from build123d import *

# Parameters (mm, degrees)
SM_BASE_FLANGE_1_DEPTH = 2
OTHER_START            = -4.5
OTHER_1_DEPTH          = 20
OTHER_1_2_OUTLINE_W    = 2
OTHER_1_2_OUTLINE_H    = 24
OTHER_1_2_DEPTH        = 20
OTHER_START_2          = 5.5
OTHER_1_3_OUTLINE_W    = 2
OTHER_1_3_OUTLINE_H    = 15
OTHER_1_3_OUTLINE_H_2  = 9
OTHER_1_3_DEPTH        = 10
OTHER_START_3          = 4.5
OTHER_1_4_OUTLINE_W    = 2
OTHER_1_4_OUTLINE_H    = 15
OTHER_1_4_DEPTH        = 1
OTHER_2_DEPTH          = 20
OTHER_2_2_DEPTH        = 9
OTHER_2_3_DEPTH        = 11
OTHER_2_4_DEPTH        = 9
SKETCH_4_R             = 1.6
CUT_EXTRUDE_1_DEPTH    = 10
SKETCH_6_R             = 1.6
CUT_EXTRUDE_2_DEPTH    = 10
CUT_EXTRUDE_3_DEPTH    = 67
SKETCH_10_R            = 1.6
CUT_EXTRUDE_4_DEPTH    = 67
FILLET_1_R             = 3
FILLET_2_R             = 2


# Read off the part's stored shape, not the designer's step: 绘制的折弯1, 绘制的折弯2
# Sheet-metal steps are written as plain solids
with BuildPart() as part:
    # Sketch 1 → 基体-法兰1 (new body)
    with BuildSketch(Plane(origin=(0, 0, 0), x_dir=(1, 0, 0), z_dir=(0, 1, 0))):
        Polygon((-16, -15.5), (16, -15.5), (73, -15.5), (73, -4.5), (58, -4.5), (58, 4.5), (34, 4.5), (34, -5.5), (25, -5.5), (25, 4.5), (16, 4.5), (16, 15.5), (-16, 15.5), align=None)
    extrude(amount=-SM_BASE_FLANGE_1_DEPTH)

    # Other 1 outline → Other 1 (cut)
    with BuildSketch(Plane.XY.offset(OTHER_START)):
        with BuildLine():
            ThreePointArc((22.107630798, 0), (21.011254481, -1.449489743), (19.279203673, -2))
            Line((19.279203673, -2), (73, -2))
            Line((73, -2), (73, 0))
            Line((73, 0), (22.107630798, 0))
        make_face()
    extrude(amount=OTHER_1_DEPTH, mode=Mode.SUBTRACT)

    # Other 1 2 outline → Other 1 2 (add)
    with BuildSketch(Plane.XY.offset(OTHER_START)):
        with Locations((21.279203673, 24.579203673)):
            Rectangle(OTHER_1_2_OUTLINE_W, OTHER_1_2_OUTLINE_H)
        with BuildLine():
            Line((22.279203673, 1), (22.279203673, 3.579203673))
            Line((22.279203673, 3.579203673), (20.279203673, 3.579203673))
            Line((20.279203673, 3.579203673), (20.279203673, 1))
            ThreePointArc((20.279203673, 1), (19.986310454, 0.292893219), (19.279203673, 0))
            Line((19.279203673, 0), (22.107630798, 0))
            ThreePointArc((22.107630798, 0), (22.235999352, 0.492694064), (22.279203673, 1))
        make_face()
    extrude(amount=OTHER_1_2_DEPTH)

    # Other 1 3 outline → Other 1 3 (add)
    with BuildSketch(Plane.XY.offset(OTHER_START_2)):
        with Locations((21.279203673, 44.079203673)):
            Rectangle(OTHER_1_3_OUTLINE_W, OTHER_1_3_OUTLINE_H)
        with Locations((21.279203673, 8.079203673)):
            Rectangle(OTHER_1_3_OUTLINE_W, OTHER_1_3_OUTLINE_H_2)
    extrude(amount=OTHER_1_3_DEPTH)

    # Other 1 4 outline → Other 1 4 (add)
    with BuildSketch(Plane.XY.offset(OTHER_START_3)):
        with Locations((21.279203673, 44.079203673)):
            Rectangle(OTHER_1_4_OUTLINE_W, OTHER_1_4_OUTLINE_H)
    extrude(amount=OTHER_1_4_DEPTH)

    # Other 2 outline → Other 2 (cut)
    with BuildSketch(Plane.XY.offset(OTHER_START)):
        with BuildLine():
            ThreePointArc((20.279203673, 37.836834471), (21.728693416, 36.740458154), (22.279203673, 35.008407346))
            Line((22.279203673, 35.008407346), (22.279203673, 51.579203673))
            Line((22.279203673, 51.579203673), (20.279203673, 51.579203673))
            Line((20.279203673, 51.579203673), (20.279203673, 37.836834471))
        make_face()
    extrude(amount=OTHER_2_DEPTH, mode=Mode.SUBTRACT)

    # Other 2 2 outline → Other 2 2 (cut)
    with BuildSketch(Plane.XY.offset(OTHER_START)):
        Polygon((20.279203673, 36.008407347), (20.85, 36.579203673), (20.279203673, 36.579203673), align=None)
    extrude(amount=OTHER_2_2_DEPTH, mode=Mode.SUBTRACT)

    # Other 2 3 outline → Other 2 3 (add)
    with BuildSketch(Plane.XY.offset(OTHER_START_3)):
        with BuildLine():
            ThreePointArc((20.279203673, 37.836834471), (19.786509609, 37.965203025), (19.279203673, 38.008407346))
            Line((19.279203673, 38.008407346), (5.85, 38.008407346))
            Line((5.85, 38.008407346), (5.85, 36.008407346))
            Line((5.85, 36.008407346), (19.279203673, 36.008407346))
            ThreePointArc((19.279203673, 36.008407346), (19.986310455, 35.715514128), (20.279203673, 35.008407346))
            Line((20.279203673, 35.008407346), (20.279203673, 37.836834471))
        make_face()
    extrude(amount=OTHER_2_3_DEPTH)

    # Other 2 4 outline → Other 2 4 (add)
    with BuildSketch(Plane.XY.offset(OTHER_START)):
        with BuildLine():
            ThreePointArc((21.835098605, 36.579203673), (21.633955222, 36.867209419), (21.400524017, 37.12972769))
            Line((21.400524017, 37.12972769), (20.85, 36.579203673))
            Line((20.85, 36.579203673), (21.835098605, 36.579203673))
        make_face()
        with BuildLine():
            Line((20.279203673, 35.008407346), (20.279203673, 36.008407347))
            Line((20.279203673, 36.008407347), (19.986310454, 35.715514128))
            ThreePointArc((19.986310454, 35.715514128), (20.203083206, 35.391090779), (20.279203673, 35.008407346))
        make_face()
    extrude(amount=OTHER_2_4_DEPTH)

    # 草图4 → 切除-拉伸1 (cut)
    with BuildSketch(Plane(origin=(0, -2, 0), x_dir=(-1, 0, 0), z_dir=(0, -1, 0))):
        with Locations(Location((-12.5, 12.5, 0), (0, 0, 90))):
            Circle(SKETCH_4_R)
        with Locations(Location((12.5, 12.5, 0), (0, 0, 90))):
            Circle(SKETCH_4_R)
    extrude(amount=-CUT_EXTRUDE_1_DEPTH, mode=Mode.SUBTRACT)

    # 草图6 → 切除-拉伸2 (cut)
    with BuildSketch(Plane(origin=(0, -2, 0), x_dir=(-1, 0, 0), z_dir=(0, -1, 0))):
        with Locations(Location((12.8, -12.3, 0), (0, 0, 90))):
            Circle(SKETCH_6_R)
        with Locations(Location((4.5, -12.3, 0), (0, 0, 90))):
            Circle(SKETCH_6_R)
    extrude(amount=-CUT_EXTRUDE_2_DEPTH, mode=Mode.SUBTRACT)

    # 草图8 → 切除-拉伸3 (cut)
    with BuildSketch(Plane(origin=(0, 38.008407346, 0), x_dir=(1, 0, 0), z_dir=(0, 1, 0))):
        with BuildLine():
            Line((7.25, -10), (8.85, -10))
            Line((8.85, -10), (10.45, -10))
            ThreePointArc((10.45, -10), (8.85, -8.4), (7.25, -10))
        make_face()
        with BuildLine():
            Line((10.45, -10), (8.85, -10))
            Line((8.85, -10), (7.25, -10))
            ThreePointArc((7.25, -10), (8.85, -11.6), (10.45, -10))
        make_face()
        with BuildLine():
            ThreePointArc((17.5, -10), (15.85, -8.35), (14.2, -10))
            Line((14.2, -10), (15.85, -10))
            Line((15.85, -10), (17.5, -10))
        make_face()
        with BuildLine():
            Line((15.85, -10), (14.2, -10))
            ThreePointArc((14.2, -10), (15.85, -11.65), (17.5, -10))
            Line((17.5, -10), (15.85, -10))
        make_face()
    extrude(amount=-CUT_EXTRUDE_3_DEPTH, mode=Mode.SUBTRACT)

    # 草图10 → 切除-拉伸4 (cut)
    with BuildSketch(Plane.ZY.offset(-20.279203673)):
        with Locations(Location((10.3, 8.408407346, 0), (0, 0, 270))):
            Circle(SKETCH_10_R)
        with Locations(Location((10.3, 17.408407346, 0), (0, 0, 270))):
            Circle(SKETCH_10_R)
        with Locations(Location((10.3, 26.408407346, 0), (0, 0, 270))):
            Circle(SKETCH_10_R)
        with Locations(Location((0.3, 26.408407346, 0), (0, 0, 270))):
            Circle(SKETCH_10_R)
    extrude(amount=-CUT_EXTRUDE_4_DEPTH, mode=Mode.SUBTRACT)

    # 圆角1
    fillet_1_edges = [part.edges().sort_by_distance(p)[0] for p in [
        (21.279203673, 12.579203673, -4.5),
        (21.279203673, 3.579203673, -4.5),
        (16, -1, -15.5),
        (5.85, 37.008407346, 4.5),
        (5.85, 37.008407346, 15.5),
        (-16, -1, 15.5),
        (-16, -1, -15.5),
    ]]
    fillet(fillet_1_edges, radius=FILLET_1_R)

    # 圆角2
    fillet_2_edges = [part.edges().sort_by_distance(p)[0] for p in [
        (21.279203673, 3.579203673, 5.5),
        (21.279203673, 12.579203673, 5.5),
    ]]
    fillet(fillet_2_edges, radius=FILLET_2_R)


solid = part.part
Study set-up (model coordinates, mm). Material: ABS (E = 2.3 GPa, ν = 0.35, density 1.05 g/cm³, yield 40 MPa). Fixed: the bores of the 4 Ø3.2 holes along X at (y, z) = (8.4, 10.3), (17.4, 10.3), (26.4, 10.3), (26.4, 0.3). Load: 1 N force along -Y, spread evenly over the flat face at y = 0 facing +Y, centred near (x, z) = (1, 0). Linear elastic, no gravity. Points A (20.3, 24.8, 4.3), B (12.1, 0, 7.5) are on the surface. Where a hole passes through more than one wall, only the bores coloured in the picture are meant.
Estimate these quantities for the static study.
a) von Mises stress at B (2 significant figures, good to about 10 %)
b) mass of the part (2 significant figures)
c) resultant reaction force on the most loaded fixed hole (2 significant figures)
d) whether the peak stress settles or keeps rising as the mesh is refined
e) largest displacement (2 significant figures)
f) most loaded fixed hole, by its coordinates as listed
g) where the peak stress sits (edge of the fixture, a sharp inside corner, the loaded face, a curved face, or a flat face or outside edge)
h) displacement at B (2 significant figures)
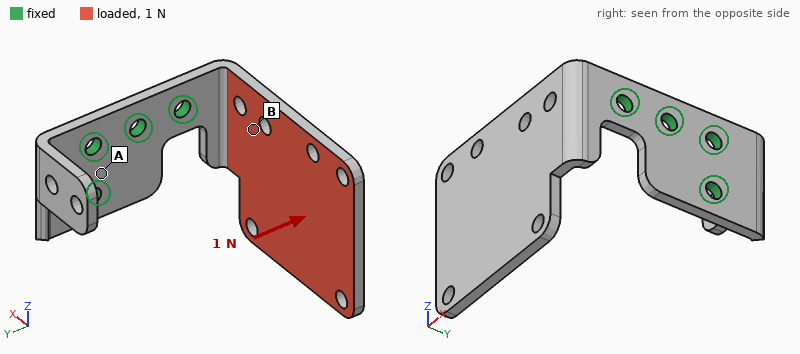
0.78 MPa
3.8 g
1.0 N
keeps rising
0.66 mm
(8.4, 10.3)
edge of the fixture
0.12 mm
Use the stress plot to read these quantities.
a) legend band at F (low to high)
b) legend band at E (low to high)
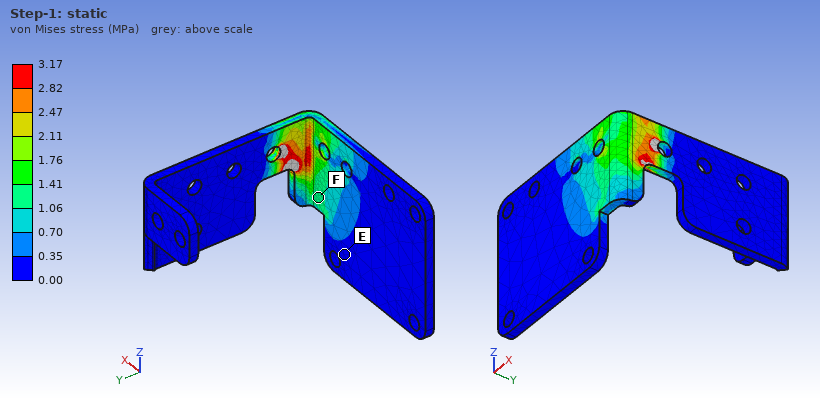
1.06 to 1.41 MPa
0.00 to 0.35 MPa
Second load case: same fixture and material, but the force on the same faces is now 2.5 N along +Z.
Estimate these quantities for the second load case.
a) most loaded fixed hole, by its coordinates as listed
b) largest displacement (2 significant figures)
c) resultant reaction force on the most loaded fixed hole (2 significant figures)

(8.4, 10.3)
0.68 mm
3.4 N
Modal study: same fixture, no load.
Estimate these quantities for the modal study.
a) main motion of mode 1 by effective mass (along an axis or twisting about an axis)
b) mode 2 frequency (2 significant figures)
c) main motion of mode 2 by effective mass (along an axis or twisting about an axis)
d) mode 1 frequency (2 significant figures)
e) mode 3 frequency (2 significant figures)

along Y
250 Hz
along Z
170 Hz
680 Hz
